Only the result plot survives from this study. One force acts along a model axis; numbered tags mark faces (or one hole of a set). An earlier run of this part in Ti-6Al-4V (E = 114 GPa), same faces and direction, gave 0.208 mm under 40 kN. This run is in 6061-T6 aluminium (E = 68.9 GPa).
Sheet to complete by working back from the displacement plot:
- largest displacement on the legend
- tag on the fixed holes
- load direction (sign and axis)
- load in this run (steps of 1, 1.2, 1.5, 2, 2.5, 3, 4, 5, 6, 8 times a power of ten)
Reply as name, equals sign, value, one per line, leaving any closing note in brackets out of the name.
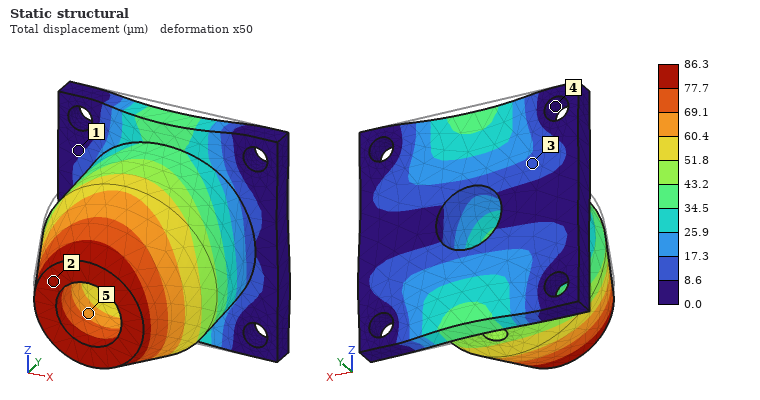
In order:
largest displacement on the legend = 86.3 µm
tag on the fixed holes = 4
load direction = -Z
load in this run = 10 kN
